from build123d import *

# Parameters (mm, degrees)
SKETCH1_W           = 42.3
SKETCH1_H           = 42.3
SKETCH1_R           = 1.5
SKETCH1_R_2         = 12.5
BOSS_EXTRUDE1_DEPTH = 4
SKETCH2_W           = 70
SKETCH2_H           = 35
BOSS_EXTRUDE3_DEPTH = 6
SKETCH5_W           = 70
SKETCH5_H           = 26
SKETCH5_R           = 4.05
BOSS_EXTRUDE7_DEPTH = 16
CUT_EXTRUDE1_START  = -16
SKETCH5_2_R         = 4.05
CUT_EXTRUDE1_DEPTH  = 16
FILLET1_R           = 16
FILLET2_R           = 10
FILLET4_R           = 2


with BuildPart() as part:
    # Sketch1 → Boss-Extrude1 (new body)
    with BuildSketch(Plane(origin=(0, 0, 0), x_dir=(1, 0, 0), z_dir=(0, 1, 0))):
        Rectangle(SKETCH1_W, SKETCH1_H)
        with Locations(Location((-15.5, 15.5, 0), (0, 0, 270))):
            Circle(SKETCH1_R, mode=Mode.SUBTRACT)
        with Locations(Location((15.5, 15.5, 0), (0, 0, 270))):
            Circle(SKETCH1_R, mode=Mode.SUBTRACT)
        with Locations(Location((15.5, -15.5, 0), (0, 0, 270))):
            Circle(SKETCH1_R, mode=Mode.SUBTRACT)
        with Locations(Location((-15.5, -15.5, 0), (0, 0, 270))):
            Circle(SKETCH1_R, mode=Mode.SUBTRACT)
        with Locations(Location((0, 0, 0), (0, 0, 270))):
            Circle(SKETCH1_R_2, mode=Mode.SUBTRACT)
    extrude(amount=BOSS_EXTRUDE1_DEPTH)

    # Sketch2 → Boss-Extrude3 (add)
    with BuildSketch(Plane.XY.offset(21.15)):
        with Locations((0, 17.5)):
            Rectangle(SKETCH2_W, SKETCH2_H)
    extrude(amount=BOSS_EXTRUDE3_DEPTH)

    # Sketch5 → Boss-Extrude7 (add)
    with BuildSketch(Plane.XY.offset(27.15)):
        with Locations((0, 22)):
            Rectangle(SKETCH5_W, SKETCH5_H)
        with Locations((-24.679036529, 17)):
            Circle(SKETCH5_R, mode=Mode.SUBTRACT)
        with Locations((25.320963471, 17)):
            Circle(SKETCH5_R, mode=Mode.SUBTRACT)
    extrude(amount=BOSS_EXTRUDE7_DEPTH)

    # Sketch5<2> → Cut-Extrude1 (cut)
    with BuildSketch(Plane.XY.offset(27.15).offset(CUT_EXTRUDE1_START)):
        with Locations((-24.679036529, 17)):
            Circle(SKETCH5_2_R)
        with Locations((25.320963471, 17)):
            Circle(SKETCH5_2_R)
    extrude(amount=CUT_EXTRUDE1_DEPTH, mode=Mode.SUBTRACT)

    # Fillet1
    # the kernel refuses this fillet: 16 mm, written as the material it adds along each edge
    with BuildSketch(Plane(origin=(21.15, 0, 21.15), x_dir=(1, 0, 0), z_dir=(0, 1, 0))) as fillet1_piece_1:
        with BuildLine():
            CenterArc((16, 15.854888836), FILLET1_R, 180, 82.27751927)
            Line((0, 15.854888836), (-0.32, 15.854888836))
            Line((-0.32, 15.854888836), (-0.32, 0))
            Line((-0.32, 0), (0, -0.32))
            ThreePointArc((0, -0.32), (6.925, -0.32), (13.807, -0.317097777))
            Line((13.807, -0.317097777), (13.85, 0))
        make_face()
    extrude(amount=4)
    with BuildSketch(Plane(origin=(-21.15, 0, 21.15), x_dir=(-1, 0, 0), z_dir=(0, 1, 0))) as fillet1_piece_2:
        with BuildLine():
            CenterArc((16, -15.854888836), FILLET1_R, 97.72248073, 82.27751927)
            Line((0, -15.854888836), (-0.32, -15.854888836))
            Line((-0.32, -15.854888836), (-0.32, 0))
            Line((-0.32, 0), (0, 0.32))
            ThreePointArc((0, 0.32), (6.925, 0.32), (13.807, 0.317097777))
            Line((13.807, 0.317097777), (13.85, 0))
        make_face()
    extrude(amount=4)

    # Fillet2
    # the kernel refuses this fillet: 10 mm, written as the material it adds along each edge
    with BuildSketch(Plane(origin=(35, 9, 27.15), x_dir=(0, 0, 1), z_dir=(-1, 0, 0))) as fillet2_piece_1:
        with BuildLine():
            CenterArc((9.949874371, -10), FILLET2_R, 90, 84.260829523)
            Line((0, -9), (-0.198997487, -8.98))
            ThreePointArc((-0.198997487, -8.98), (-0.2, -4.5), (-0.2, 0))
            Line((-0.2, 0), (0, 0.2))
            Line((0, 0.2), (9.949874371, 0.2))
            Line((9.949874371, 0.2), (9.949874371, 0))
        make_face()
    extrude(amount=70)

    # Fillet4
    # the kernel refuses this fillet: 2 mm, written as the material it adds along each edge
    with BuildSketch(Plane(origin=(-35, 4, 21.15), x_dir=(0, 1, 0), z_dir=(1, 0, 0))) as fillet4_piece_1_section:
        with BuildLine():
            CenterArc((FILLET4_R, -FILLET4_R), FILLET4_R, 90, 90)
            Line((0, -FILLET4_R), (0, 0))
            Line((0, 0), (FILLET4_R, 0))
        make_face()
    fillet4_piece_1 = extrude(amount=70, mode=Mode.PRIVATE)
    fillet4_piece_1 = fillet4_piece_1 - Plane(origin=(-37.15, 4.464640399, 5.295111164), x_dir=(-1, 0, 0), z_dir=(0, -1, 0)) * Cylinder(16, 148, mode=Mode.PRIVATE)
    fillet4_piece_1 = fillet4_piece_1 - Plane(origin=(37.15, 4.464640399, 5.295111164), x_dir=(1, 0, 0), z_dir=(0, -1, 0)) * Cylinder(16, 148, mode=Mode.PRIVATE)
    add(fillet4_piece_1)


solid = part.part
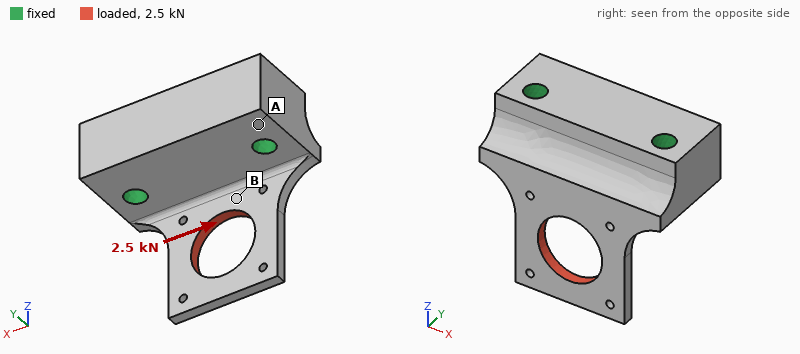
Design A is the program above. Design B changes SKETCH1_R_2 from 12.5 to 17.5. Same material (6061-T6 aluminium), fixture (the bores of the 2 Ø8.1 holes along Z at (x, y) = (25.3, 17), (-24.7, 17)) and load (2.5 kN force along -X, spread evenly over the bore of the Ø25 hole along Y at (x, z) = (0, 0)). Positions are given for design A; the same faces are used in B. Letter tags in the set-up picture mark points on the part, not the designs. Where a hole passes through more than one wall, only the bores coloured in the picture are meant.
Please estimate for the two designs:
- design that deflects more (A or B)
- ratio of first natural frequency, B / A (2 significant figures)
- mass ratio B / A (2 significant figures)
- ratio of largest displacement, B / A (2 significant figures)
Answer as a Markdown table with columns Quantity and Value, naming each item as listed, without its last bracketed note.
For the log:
| Quantity | Value |
|---|---|
| design that deflects more | B |
| ratio of first natural frequency, B / A | 0.86 |
| mass ratio B / A | 0.96 |
| ratio of largest displacement, B / A | 4.3 |
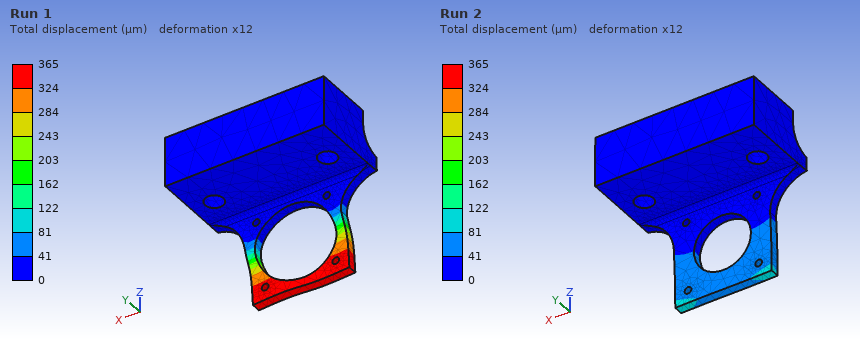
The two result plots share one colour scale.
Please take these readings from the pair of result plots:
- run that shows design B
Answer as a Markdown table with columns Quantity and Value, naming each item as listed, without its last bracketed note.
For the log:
| Quantity | Value |
|---|---|
| run that shows design B | Run 1 |
